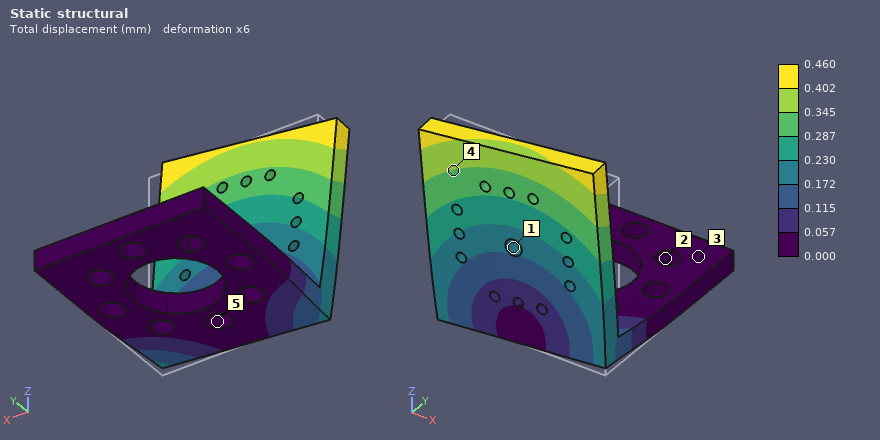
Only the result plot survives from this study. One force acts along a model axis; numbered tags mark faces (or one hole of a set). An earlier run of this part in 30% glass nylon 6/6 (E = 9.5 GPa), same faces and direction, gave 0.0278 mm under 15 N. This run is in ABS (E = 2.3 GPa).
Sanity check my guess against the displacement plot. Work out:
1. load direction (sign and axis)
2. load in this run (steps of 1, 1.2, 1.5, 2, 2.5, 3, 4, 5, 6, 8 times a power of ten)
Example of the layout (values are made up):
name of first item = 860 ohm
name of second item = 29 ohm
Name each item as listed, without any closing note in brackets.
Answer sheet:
load direction = -X
load in this run = 60 N
